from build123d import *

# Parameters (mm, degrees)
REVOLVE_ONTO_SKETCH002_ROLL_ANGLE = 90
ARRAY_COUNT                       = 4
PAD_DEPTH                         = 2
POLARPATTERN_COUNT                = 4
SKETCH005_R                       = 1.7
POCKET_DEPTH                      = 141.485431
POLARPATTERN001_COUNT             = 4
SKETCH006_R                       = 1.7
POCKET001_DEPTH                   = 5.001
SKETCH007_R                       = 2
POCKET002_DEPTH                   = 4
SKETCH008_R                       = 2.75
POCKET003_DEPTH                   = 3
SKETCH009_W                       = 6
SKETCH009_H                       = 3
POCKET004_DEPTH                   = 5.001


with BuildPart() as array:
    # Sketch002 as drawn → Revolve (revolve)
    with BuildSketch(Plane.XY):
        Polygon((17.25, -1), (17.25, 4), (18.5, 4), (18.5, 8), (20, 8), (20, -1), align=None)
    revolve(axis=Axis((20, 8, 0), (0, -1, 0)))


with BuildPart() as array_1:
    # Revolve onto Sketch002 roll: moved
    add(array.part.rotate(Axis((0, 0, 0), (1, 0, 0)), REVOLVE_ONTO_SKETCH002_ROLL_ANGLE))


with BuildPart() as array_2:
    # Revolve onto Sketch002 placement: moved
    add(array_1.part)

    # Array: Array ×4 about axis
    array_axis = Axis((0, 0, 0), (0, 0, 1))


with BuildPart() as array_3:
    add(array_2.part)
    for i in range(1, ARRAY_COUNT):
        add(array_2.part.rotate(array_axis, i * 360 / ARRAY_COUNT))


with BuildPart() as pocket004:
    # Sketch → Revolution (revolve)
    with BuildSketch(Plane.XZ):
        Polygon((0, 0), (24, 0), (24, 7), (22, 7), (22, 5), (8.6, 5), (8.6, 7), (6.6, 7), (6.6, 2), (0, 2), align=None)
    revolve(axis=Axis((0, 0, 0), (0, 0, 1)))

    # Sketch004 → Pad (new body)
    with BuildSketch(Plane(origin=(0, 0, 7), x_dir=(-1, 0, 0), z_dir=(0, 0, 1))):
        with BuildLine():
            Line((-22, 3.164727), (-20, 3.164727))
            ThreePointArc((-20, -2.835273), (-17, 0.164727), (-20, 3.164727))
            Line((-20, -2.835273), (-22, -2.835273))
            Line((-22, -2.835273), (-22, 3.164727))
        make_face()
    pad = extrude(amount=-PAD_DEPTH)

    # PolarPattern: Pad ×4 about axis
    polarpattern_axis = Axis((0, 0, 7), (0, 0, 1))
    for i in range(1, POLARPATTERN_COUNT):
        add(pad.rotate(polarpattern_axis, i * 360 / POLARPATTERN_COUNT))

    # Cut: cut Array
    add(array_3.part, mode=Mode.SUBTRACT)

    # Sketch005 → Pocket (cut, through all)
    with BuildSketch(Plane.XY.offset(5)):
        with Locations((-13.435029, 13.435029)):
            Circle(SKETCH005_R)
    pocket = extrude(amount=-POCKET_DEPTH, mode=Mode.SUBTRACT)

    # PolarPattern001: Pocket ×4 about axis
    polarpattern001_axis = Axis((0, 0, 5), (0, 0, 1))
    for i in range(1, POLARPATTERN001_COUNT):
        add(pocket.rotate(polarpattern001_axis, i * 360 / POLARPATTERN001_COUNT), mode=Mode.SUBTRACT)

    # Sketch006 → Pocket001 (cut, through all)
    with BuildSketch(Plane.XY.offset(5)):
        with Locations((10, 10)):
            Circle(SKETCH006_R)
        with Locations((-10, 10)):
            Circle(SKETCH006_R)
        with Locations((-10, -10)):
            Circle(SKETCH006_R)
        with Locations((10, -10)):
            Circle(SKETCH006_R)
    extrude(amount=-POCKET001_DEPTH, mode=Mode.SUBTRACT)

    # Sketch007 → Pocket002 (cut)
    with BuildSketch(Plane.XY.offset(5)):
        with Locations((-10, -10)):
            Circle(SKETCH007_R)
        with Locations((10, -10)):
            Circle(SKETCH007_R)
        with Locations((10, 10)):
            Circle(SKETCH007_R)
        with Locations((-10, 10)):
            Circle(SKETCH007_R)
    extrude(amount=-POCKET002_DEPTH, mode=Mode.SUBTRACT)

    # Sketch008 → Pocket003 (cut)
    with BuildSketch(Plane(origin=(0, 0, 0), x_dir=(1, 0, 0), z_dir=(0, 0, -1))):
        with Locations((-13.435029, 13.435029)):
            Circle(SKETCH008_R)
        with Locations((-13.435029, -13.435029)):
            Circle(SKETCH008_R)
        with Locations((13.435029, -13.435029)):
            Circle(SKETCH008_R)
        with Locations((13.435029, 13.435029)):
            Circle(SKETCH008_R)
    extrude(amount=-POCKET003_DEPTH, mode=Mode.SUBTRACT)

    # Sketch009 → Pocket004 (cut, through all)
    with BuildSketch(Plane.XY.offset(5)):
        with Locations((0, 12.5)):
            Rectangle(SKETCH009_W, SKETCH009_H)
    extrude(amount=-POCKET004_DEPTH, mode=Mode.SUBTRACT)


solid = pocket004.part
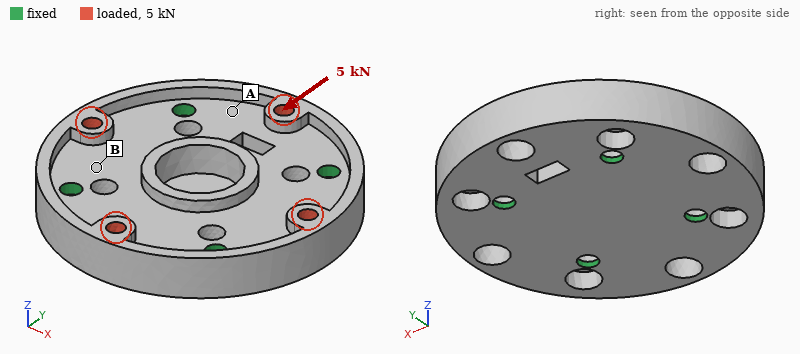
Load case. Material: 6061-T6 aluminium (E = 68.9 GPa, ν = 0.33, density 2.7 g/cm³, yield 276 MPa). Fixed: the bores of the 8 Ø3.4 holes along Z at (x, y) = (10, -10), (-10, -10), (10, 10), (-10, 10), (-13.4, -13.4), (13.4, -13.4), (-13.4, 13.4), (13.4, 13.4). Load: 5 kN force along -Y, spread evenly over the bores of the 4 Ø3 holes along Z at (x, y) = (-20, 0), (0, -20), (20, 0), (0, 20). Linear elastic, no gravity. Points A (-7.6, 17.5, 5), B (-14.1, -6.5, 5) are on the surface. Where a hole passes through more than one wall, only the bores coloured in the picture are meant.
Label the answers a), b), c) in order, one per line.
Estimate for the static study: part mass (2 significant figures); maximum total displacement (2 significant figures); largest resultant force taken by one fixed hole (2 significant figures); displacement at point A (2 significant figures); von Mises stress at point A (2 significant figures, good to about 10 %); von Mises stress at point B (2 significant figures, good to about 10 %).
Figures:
a) 23 g
b) 31 µm
c) 920 N
d) 7.2 µm
e) 42 MPa
f) 20 MPa
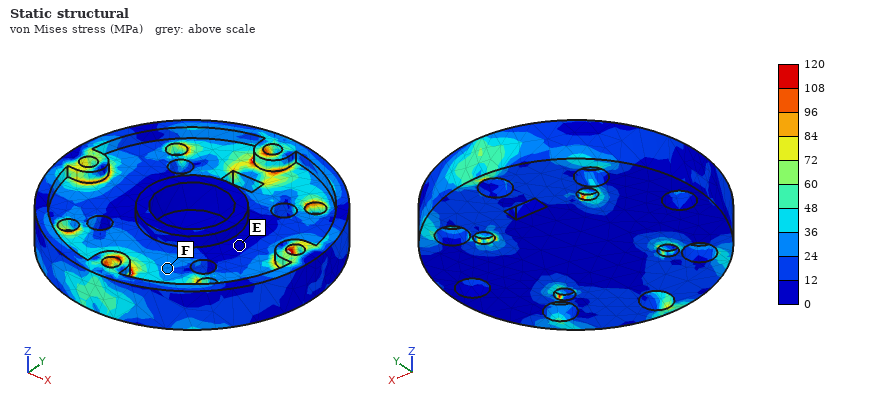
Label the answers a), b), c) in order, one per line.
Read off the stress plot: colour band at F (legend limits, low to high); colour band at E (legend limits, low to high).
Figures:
a) 24 to 36 MPa
b) 0 to 12 MPa
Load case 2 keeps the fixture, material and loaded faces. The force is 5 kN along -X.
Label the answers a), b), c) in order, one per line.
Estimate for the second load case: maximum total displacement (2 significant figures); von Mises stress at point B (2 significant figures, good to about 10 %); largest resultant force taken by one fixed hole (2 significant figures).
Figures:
a) 28 µm
b) 27 MPa
c) 910 N
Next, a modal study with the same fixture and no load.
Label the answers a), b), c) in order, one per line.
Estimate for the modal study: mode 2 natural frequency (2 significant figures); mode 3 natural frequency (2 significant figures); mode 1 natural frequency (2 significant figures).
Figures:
a) 21 kHz
b) 21 kHz
c) 19 kHz
